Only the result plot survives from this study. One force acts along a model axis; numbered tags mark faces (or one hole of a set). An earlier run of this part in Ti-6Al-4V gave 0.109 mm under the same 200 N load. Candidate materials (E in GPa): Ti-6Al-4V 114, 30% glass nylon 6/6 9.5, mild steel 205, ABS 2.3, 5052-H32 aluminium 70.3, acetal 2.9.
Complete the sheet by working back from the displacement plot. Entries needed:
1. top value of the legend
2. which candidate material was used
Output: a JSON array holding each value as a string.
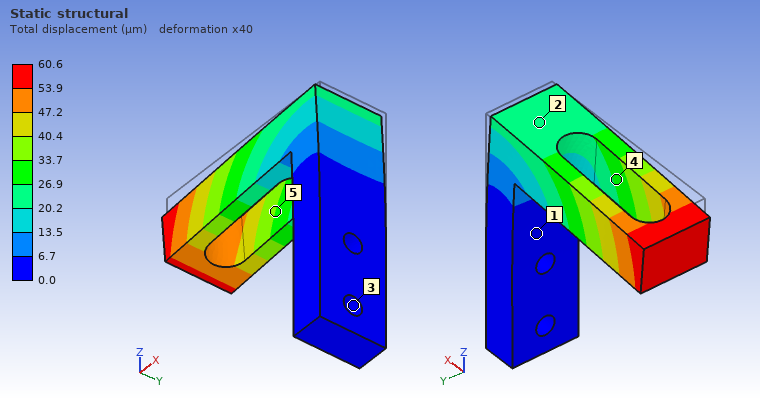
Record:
["60.6 µm", "mild steel"]
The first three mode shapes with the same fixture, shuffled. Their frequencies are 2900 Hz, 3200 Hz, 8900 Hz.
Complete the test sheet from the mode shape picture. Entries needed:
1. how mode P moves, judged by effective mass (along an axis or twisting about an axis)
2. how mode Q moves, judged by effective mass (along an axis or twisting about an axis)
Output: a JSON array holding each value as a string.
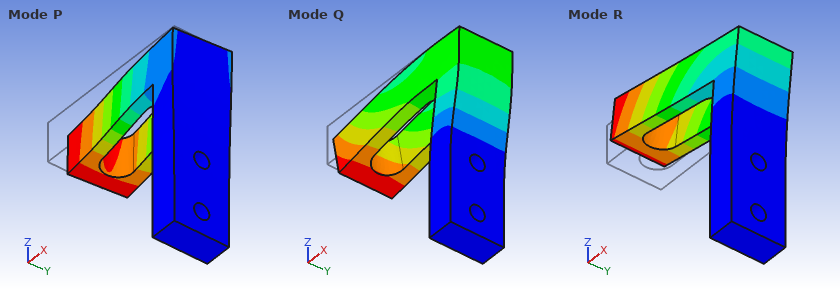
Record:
["along Y", "along X"]
